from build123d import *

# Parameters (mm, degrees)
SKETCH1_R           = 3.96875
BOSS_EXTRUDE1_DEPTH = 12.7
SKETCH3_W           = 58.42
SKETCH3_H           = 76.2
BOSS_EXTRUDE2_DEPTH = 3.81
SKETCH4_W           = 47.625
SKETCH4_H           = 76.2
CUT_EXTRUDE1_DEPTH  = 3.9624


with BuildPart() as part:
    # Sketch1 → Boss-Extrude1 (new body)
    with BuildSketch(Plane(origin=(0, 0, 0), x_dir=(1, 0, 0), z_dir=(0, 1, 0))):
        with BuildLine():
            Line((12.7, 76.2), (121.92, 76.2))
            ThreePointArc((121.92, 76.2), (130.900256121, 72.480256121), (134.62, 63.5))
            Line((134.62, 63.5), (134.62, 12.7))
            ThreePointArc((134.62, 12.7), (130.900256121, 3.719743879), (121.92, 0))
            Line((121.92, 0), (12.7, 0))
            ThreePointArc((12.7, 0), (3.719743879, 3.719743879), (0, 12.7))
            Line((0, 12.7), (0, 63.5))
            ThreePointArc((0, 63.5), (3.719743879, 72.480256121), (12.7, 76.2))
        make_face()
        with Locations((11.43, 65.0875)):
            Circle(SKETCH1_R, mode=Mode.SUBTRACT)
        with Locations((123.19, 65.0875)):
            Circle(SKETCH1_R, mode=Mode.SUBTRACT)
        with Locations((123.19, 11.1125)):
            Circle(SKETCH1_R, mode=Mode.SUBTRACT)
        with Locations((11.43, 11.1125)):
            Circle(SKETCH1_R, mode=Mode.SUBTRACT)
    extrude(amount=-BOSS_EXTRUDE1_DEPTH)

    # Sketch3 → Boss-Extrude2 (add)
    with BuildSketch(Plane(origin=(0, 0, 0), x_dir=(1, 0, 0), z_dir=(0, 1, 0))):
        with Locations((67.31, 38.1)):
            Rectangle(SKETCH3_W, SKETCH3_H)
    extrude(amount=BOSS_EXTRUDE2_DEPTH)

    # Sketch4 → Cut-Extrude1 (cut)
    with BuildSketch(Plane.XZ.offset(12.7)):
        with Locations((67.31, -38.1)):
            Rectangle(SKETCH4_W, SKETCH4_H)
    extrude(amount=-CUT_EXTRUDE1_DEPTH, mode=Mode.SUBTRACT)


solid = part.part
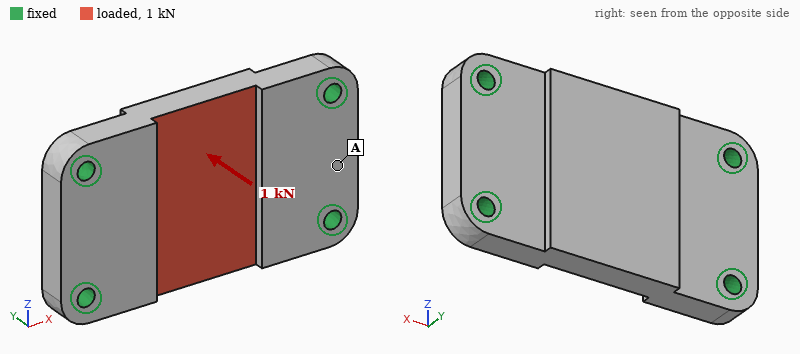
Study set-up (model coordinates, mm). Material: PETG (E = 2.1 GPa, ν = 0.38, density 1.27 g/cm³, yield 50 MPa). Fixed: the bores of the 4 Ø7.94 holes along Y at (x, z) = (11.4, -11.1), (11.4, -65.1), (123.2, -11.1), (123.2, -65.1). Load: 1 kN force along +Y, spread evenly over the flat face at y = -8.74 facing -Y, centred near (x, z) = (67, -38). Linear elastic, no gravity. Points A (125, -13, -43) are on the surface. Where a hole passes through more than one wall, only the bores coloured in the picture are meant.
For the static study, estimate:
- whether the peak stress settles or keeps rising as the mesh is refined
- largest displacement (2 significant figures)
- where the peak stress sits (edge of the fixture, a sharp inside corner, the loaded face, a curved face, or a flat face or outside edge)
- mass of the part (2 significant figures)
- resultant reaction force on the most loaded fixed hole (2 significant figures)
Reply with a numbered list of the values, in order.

1. keeps rising
2. 0.26 mm
3. edge of the fixture
4. 160 g
5. 400 N
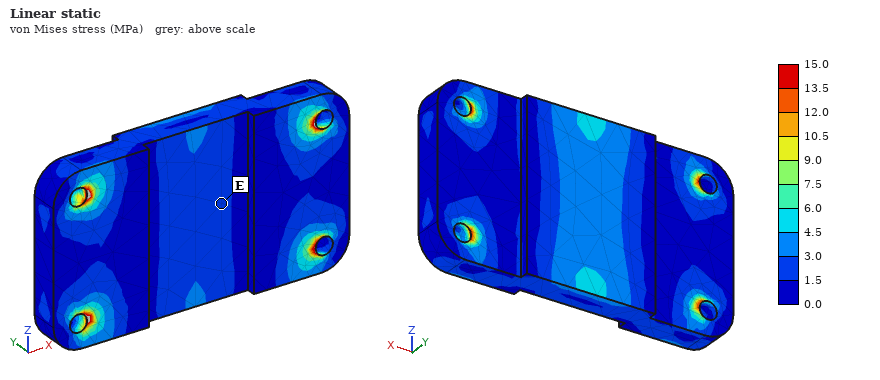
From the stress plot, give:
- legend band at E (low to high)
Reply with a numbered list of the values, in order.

1. 1.5 to 3.0 MPa
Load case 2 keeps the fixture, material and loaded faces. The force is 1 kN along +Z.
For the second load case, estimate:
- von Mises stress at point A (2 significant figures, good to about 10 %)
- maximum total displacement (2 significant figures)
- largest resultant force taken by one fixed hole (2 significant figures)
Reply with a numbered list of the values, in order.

1. 0.43 MPa
2. 64 µm
3. 310 N
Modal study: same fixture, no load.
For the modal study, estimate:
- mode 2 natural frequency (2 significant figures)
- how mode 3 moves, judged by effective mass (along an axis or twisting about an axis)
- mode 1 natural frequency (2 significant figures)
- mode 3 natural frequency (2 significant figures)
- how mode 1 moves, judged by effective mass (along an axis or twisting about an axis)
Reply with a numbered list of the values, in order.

1. 1700 Hz
2. twisting about Z
3. 1200 Hz
4. 2800 Hz
5. along Y
